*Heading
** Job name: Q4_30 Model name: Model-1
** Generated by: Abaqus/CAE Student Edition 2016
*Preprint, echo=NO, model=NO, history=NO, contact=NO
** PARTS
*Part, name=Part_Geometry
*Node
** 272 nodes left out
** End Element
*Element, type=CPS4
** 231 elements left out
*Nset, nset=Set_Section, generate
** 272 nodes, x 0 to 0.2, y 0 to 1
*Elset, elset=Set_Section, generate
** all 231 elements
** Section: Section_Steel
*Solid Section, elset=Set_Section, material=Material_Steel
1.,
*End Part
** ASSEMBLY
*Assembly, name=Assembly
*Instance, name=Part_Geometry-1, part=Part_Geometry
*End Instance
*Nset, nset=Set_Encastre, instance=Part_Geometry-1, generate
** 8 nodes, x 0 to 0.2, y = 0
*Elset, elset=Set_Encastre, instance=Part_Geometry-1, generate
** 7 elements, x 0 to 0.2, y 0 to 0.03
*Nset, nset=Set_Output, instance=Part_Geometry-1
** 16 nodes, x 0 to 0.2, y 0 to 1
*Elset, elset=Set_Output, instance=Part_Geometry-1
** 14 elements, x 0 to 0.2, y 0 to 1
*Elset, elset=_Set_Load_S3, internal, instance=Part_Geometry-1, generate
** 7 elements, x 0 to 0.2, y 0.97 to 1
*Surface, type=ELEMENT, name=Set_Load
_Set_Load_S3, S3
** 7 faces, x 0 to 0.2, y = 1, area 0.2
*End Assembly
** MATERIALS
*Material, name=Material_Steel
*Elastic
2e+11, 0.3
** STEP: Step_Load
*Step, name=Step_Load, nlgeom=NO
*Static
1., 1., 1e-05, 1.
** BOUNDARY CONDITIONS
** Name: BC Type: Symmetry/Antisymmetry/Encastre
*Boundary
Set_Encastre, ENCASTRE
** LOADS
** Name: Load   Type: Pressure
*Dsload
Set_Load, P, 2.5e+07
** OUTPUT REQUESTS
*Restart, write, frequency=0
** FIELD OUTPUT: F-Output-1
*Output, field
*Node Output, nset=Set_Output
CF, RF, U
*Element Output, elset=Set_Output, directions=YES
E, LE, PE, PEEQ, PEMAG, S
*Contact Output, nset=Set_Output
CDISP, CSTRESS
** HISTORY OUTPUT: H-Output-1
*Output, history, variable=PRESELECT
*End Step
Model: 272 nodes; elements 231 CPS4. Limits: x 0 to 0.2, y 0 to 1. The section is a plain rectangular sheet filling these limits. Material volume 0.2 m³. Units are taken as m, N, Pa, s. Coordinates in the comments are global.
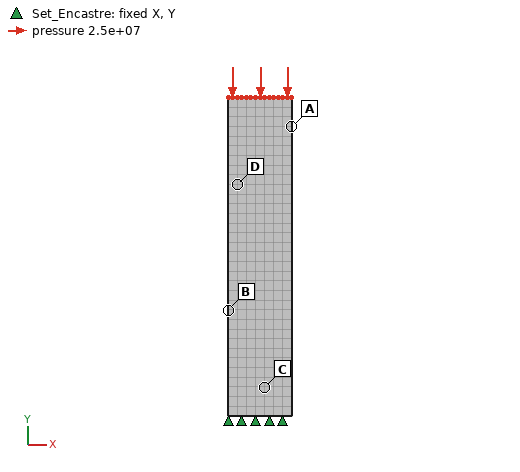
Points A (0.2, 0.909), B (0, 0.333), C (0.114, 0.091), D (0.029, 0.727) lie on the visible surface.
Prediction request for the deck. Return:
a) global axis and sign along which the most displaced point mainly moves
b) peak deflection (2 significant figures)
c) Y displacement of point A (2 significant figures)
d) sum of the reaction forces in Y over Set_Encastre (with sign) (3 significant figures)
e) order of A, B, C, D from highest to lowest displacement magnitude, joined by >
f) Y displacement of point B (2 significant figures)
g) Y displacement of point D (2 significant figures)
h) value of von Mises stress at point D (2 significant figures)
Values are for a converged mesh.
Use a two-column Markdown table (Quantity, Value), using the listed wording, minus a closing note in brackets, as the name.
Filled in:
| Quantity | Value |
|---|---|
| global axis and sign along which the most displaced point mainly moves | -Y |
| peak deflection | 1.2e-04 m |
| Y displacement of point A | -1.1e-04 m |
| sum of the reaction forces in Y over Set_Encastre (with sign) | 5.00e+06 N |
| order of A, B, C, D from highest to lowest displacement magnitude, joined by > | A > D > B > C |
| Y displacement of point B | -4.1e-05 m |
| Y displacement of point D | -9.1e-05 m |
| value of von Mises stress at point D | 2.5e+07 Pa |
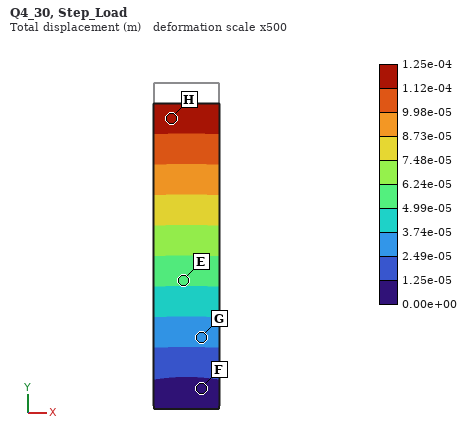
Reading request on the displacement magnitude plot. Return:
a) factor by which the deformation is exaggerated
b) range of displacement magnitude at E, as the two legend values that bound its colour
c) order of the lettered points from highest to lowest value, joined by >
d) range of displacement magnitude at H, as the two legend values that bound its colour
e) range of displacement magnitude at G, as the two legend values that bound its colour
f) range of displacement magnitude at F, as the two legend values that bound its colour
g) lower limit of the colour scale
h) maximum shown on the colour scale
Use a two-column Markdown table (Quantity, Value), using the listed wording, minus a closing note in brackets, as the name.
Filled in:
| Quantity | Value |
|---|---|
| factor by which the deformation is exaggerated | 500 |
| range of displacement magnitude at E, as the two legend values that bound its colour | 4.99e-05 to 6.24e-05 m |
| order of the lettered points from highest to lowest value, joined by > | H > E > G > F |
| range of displacement magnitude at H, as the two legend values that bound its colour | 1.12e-04 to 1.25e-04 m |
| range of displacement magnitude at G, as the two legend values that bound its colour | 2.49e-05 to 3.74e-05 m |
| range of displacement magnitude at F, as the two legend values that bound its colour | 0.00e+00 to 1.25e-05 m |
| lower limit of the colour scale | 0.00e+00 m |
| maximum shown on the colour scale | 1.25e-04 m |
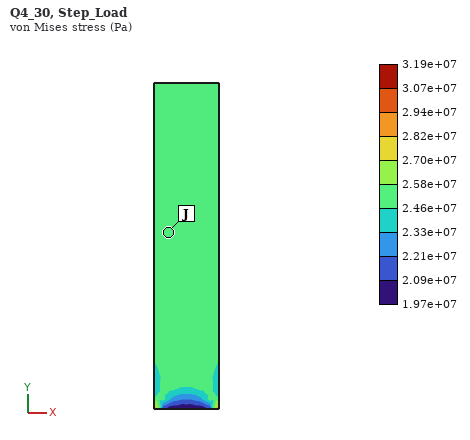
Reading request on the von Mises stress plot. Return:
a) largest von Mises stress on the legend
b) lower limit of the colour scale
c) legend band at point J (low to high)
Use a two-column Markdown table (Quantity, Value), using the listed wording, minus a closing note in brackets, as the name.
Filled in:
| Quantity | Value |
|---|---|
| largest von Mises stress on the legend | 3.19e+07 Pa |
| lower limit of the colour scale | 1.97e+07 Pa |
| legend band at point J | 2.46e+07 to 2.58e+07 Pa |
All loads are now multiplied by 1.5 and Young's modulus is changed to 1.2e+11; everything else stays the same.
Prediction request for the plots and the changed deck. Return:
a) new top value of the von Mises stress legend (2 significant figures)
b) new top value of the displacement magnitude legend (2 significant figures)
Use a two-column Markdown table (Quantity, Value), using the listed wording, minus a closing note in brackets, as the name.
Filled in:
| Quantity | Value |
|---|---|
| new top value of the von Mises stress legend | 4.8e+07 Pa |
| new top value of the displacement magnitude legend | 3.1e-04 m |
